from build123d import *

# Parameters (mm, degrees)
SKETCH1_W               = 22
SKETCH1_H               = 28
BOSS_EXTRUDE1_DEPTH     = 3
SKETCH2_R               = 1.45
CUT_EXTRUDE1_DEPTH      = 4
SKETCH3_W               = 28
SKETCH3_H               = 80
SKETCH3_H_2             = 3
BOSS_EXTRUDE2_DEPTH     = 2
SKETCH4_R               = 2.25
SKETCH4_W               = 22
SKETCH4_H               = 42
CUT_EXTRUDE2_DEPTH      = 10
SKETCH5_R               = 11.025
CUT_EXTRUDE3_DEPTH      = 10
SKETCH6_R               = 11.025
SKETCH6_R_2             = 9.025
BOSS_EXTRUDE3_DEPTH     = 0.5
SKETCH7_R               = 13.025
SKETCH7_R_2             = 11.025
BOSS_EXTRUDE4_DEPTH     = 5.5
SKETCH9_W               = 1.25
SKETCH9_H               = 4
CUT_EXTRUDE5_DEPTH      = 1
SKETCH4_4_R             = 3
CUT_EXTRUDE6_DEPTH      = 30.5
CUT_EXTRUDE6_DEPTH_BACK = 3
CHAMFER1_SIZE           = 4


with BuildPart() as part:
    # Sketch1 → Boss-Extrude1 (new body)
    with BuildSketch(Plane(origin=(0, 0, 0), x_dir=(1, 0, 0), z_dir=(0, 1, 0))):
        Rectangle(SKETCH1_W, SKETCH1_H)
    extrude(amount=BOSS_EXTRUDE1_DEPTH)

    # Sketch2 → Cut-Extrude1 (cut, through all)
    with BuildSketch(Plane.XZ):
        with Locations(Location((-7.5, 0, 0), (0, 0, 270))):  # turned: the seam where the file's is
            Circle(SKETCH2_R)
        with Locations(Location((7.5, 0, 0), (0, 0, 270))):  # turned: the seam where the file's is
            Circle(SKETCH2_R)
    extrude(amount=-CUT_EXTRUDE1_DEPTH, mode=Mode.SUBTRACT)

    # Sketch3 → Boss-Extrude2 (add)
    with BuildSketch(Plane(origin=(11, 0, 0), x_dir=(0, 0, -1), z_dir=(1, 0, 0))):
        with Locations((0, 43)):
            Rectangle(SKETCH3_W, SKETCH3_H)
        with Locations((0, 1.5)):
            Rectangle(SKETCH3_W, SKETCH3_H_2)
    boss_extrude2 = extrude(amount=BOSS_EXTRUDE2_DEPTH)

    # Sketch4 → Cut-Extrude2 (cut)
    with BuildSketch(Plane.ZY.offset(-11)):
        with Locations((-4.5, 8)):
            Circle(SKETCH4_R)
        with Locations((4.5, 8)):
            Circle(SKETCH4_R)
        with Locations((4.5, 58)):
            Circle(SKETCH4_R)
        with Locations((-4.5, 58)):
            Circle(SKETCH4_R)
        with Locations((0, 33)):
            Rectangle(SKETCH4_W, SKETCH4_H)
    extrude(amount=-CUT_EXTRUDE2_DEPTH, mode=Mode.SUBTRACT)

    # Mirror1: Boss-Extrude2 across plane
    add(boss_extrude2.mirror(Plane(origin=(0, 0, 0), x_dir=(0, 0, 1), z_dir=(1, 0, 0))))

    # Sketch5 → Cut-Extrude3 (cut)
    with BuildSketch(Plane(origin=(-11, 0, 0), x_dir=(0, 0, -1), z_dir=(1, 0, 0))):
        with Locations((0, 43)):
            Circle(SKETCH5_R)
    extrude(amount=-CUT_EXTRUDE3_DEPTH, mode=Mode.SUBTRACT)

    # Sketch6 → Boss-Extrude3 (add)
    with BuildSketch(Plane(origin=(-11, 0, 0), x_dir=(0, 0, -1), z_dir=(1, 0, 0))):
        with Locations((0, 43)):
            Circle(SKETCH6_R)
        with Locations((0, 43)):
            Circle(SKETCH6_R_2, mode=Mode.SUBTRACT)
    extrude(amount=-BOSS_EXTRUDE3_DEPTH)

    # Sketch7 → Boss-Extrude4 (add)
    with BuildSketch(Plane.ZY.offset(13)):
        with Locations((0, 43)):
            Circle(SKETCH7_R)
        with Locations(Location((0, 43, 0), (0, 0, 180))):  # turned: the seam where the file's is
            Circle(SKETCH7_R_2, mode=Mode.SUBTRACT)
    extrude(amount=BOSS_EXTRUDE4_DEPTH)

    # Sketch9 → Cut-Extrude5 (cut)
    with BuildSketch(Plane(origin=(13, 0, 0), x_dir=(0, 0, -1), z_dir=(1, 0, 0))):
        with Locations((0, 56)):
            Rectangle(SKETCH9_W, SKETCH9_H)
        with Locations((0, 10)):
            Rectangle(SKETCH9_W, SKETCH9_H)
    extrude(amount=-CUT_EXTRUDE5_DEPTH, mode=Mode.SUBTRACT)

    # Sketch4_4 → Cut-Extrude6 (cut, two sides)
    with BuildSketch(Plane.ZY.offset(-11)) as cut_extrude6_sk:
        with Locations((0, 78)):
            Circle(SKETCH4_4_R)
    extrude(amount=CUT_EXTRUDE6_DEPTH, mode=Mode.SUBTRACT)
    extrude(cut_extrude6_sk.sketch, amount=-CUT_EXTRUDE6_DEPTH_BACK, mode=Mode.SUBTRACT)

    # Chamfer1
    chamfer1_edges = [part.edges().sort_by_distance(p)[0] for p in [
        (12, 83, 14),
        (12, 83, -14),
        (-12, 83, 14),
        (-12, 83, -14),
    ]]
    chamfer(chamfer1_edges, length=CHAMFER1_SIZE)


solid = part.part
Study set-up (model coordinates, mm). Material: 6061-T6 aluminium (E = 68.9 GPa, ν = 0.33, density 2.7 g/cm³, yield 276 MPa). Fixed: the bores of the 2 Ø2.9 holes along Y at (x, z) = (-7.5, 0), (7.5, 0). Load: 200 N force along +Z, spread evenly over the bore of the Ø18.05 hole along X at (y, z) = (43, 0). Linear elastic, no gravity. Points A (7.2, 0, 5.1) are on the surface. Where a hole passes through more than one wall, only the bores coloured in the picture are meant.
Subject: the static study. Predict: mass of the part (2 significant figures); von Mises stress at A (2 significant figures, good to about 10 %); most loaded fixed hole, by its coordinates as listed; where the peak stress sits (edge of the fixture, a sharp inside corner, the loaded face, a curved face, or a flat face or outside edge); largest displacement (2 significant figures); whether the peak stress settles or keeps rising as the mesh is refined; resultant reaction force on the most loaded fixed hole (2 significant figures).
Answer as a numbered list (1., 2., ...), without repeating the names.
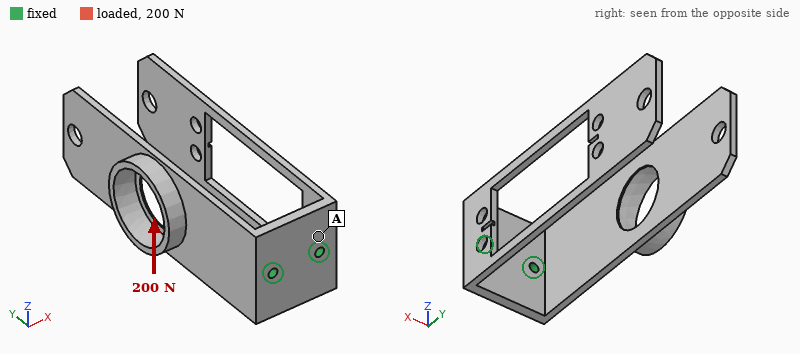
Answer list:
1. 24 g
2. 29 MPa
3. (-7.5, 0)
4. edge of the fixture
5. 0.72 mm
6. keeps rising
7. 230 N
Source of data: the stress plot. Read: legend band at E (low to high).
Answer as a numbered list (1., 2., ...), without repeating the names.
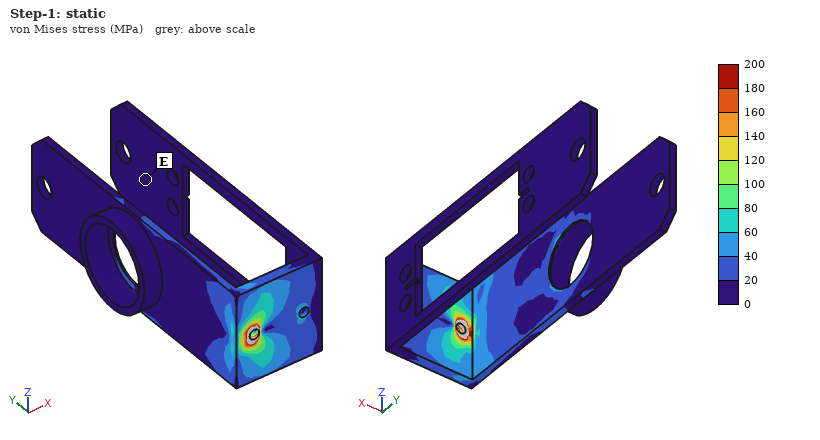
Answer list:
1. 0 to 20 MPa
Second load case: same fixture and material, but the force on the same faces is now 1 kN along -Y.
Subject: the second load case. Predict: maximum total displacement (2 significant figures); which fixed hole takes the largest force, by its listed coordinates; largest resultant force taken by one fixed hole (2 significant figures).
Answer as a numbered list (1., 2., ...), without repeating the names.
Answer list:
1. 1.0 mm
2. (-7.5, 0)
3. 1.1 kN
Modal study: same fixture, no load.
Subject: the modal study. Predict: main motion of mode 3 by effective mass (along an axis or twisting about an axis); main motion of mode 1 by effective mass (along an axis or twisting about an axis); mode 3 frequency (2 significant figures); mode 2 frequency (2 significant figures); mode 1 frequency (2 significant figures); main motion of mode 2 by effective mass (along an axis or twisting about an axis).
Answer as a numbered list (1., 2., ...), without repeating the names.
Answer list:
1. along Z
2. along X
3. 560 Hz
4. 260 Hz
5. 150 Hz
6. along X
